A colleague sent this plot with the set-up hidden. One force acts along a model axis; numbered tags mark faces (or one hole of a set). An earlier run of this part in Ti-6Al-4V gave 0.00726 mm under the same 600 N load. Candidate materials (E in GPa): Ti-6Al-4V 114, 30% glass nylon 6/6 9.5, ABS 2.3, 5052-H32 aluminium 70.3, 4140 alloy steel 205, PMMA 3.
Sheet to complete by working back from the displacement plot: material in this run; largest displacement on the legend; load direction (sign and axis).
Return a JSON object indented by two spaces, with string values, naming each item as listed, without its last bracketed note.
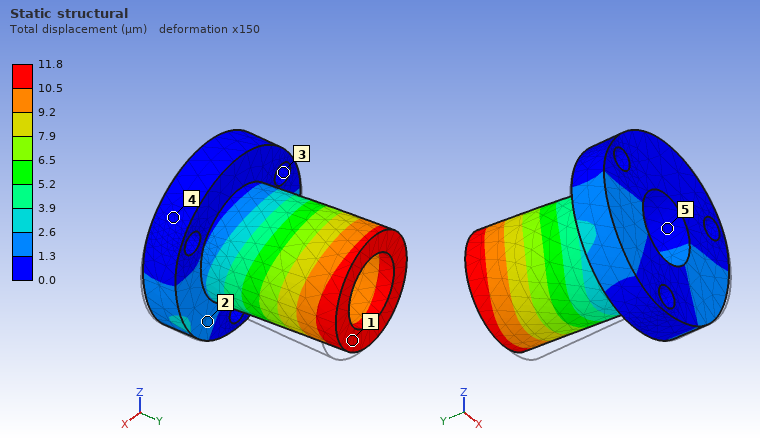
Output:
{
  "material in this run": "5052-H32 aluminium",
  "largest displacement on the legend": "11.8 µm",
  "load direction": "-X"
}
